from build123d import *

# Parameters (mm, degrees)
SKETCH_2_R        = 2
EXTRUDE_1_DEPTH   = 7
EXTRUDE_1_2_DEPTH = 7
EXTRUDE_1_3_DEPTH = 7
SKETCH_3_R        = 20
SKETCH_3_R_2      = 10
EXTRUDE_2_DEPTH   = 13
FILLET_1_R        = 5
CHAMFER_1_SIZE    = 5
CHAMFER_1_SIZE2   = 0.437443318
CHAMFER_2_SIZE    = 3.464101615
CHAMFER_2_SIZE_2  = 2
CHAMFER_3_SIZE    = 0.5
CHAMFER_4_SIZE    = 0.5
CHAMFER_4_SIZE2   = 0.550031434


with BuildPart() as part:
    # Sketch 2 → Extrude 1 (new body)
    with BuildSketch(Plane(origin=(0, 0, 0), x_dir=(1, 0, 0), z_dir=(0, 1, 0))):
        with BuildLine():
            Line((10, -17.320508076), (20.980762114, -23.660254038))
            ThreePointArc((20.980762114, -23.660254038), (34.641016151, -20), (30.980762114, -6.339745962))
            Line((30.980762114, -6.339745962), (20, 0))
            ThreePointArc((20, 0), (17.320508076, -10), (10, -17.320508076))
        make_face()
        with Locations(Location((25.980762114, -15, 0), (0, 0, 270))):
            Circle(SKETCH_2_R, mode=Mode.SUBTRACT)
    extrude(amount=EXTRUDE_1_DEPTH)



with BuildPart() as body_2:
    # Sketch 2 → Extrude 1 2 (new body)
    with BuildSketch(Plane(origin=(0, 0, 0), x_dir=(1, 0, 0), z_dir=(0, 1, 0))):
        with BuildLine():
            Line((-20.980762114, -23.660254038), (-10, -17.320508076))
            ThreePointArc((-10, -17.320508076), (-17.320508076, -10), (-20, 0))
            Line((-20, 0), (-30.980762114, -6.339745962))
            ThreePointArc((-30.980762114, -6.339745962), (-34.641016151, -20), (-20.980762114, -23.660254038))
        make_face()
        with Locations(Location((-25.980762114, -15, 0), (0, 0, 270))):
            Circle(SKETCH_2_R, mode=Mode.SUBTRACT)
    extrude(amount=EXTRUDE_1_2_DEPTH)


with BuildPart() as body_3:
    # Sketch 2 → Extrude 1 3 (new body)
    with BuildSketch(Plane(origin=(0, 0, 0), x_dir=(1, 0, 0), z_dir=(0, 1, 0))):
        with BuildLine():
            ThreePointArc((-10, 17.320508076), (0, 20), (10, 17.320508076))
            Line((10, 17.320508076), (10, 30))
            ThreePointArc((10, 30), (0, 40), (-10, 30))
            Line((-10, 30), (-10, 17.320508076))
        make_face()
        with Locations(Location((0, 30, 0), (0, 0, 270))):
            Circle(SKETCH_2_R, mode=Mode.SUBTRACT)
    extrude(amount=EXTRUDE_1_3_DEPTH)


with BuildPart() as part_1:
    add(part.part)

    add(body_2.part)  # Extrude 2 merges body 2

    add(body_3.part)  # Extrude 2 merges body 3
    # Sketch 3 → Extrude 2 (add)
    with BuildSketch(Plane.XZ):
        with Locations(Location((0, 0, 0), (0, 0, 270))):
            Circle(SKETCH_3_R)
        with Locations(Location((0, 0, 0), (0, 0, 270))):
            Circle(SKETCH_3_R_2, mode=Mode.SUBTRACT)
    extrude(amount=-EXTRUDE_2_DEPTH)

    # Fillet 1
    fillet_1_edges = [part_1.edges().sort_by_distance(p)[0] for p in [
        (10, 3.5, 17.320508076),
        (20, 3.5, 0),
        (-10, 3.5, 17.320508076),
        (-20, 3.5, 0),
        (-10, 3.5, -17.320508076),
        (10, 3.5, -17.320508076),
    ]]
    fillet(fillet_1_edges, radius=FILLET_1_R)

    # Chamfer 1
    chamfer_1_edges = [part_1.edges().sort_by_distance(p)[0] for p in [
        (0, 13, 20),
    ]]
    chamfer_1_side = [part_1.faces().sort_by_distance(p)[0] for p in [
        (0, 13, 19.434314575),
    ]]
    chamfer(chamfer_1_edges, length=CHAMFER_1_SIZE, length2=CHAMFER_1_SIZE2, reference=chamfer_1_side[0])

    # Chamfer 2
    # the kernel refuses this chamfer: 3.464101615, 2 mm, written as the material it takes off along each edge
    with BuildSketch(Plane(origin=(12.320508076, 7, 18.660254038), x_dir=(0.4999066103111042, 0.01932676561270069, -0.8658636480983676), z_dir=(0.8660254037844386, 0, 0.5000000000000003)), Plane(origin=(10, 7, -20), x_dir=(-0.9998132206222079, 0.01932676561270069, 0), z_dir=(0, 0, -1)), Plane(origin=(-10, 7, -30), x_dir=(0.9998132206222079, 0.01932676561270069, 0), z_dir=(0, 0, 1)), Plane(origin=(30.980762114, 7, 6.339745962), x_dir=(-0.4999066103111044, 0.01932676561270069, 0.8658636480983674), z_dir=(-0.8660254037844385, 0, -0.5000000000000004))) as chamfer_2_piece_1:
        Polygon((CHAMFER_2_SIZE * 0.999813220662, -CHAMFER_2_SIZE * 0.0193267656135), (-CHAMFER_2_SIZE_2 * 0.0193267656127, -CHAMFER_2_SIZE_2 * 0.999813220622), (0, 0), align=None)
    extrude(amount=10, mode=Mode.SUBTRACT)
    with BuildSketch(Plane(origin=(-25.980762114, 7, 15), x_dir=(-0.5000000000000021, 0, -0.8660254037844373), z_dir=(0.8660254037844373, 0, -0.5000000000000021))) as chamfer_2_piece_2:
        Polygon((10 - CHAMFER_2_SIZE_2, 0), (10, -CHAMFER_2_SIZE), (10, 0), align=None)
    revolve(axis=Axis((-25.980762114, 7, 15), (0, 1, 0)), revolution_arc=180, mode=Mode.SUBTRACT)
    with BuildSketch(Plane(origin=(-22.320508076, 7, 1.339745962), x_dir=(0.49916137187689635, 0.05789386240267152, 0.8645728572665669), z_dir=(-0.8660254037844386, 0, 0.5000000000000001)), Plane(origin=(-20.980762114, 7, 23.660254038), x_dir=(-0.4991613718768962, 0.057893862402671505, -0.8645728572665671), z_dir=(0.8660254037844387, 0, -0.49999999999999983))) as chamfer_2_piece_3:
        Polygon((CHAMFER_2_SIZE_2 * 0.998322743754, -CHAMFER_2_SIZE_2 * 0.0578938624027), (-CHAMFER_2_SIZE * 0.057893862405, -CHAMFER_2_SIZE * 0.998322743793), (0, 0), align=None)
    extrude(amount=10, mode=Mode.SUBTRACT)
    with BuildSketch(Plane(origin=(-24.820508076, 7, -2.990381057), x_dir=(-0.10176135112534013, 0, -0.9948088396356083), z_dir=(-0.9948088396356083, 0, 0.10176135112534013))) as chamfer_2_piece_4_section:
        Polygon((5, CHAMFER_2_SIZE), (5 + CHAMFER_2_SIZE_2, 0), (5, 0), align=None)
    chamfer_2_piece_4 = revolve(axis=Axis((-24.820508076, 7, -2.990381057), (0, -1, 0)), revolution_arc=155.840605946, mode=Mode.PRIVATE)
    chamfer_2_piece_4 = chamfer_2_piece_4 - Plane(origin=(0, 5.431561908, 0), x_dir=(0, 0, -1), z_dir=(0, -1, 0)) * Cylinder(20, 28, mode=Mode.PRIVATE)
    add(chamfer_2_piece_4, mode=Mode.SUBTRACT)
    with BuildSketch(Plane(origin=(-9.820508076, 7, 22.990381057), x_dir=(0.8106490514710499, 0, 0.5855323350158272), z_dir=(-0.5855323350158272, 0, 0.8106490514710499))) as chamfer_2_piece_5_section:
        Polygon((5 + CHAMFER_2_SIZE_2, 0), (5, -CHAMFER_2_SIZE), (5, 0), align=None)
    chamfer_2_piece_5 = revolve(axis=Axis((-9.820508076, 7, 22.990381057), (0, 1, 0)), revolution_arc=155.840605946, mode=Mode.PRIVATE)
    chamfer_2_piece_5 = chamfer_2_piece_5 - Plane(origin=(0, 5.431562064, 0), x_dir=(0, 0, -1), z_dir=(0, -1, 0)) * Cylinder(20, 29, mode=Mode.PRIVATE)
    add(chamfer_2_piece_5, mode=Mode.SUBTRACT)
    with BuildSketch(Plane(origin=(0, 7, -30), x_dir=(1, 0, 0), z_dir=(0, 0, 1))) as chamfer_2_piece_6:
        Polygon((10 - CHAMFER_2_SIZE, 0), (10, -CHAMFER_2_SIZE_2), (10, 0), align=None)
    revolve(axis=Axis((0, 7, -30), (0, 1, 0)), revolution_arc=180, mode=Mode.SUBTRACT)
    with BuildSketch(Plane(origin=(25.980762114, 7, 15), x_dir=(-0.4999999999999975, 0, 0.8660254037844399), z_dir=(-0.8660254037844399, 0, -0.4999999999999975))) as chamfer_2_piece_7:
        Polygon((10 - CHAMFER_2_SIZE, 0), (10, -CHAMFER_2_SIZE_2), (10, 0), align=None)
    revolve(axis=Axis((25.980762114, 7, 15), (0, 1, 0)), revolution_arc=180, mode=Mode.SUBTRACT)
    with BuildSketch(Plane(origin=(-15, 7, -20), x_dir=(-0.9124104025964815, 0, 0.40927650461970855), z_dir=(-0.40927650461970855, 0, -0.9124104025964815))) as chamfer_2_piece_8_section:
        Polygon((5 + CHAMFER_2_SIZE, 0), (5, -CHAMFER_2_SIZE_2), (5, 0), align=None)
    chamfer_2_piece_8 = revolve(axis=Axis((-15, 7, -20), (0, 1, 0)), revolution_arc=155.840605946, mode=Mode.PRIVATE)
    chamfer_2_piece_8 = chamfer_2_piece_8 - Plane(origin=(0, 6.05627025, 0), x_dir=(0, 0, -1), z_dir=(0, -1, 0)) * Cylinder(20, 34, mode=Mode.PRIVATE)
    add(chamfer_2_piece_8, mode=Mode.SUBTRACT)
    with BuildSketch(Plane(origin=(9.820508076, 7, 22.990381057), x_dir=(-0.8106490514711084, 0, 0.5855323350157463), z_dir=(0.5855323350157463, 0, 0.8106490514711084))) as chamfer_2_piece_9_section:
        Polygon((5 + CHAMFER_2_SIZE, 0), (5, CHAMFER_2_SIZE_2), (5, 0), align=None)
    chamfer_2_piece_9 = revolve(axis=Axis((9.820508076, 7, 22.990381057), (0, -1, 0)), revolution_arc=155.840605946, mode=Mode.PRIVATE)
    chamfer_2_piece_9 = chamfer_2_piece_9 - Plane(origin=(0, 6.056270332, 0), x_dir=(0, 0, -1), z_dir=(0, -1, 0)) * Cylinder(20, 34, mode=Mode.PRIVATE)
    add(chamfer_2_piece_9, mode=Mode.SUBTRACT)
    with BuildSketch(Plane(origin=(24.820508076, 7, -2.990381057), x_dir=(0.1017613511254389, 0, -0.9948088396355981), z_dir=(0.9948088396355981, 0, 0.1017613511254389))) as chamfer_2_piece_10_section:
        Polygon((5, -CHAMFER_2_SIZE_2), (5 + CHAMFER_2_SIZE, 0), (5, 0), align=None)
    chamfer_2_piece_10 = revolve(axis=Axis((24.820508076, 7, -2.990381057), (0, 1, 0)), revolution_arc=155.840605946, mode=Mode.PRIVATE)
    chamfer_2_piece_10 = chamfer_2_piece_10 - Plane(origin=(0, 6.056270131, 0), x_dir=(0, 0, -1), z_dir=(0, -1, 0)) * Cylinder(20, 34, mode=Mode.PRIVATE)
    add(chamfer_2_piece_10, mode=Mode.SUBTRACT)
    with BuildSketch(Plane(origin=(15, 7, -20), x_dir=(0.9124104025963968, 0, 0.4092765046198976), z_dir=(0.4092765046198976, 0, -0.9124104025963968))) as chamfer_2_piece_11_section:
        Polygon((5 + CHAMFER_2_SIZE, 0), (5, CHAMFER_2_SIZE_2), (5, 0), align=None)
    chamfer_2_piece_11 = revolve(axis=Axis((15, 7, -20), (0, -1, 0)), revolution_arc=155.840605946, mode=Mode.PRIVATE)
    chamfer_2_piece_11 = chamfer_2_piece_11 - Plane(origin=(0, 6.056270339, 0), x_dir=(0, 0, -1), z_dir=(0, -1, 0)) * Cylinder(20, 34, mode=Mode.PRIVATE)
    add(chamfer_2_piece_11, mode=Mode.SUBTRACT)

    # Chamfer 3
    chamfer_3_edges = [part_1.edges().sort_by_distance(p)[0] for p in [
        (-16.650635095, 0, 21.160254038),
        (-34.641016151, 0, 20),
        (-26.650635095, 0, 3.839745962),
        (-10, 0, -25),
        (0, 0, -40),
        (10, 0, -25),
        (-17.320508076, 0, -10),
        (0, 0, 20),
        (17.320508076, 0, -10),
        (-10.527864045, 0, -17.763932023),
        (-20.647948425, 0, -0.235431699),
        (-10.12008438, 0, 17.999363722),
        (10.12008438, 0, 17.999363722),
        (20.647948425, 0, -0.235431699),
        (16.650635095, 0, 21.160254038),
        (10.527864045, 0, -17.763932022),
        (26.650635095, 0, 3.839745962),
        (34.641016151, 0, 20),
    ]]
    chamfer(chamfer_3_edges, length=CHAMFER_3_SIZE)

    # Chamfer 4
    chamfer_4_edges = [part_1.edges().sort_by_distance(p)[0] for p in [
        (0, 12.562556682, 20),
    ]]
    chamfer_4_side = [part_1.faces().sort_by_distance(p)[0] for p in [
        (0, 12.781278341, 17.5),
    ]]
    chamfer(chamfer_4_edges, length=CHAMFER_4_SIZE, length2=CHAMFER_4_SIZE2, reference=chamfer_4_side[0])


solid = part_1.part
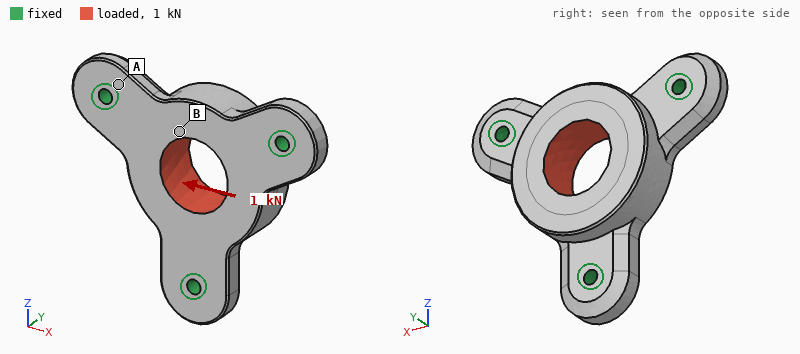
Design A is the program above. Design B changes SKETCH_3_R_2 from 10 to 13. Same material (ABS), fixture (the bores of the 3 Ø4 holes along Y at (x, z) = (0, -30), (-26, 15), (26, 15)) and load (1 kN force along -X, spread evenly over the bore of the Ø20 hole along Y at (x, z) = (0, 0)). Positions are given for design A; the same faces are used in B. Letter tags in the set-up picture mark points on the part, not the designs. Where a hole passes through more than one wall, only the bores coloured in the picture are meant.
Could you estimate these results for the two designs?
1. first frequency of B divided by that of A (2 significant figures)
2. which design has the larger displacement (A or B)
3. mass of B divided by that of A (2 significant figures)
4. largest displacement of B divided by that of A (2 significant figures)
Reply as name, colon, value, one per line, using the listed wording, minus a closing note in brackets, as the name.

first frequency of B divided by that of A: 1.1
which design has the larger displacement: B
mass of B divided by that of A: 0.85
largest displacement of B divided by that of A: 1.7
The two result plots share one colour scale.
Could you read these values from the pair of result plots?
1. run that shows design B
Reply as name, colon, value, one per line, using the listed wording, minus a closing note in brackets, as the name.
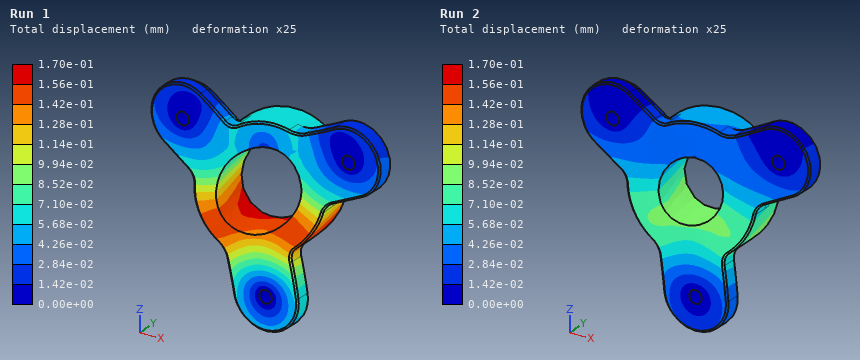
run that shows design B: Run 1
